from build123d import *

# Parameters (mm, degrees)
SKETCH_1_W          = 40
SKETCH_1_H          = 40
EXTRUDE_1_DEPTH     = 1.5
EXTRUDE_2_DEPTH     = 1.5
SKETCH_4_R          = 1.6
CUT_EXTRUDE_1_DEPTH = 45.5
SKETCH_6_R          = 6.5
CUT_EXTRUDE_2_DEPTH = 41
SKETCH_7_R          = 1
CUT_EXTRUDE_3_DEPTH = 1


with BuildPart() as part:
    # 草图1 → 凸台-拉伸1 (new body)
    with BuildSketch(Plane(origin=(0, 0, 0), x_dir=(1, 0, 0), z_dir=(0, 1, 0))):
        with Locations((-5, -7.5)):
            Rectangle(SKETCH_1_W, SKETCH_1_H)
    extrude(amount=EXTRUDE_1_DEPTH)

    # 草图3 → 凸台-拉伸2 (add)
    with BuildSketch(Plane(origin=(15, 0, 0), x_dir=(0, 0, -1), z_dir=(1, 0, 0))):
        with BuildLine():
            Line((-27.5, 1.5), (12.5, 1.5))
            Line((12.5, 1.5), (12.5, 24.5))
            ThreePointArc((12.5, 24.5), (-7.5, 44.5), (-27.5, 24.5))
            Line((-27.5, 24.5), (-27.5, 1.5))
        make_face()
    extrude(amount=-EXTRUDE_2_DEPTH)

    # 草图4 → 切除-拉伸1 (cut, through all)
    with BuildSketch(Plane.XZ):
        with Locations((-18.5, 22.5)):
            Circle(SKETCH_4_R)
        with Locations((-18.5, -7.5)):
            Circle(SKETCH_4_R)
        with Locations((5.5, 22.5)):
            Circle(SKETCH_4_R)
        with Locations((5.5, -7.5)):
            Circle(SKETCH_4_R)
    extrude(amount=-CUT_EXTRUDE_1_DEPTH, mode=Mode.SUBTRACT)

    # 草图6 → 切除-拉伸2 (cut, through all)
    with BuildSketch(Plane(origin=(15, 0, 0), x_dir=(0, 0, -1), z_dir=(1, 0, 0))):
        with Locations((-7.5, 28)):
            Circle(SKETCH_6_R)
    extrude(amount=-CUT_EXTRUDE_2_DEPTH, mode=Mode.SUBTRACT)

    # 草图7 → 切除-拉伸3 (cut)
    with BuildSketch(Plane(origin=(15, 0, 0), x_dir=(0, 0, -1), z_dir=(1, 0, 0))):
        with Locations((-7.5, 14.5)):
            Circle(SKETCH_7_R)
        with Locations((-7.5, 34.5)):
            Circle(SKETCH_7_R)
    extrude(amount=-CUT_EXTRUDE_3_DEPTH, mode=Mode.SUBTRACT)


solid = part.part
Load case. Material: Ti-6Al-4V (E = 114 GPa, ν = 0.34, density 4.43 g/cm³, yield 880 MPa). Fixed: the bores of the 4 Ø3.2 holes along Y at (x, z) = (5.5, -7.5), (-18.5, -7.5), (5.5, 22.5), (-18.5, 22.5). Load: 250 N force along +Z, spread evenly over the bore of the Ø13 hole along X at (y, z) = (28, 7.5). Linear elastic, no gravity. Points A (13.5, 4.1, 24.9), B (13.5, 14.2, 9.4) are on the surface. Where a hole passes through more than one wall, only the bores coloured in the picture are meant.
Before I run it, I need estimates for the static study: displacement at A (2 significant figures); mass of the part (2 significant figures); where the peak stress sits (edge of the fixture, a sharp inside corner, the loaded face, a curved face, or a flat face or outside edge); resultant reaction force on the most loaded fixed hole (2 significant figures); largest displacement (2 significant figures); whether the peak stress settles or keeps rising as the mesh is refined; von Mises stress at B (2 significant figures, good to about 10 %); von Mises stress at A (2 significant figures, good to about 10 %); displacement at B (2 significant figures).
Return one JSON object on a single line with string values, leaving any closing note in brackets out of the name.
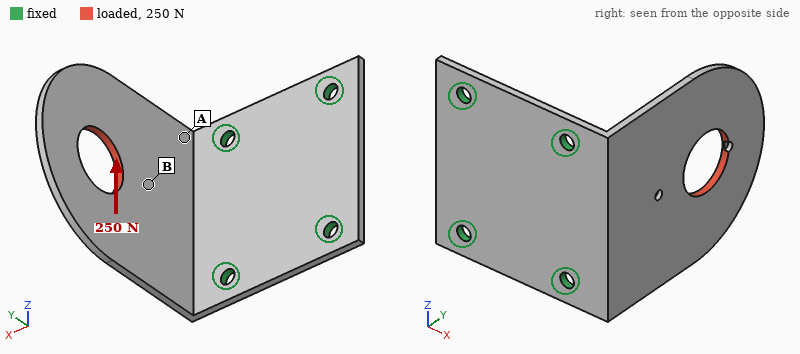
{"displacement at A": "0.069 mm", "mass of the part": "20 g", "where the peak stress sits": "edge of the fixture", "resultant reaction force on the most loaded fixed hole": "260 N", "largest displacement": "0.19 mm", "whether the peak stress settles or keeps rising as the mesh is refined": "keeps rising", "von Mises stress at B": "32 MPa", "von Mises stress at A": "89 MPa", "displacement at B": "0.058 mm"}
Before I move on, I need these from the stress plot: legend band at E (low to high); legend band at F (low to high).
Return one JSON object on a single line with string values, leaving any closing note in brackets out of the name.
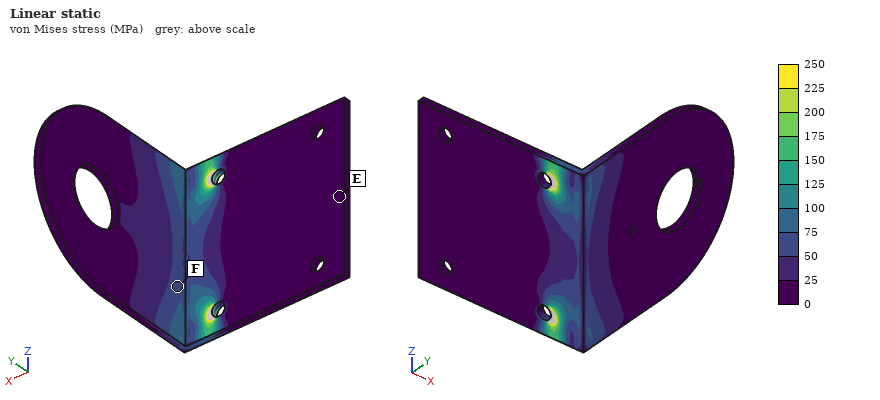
{"legend band at E": "0 to 25 MPa", "legend band at F": "50 to 75 MPa"}
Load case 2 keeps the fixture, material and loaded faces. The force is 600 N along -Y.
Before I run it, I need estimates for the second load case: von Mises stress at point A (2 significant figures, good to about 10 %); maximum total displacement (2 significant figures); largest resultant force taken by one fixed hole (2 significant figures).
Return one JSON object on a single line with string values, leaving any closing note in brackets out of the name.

{"von Mises stress at point A": "47 MPa", "maximum total displacement": "0.74 mm", "largest resultant force taken by one fixed hole": "320 N"}
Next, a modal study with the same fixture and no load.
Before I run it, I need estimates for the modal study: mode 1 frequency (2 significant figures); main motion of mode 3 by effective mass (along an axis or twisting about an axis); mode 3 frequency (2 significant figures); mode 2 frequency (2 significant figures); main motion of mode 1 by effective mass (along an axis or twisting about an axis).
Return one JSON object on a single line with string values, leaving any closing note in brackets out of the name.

{"mode 1 frequency": "620 Hz", "main motion of mode 3 by effective mass": "along Z", "mode 3 frequency": "2900 Hz", "mode 2 frequency": "1800 Hz", "main motion of mode 1 by effective mass": "along X"}
